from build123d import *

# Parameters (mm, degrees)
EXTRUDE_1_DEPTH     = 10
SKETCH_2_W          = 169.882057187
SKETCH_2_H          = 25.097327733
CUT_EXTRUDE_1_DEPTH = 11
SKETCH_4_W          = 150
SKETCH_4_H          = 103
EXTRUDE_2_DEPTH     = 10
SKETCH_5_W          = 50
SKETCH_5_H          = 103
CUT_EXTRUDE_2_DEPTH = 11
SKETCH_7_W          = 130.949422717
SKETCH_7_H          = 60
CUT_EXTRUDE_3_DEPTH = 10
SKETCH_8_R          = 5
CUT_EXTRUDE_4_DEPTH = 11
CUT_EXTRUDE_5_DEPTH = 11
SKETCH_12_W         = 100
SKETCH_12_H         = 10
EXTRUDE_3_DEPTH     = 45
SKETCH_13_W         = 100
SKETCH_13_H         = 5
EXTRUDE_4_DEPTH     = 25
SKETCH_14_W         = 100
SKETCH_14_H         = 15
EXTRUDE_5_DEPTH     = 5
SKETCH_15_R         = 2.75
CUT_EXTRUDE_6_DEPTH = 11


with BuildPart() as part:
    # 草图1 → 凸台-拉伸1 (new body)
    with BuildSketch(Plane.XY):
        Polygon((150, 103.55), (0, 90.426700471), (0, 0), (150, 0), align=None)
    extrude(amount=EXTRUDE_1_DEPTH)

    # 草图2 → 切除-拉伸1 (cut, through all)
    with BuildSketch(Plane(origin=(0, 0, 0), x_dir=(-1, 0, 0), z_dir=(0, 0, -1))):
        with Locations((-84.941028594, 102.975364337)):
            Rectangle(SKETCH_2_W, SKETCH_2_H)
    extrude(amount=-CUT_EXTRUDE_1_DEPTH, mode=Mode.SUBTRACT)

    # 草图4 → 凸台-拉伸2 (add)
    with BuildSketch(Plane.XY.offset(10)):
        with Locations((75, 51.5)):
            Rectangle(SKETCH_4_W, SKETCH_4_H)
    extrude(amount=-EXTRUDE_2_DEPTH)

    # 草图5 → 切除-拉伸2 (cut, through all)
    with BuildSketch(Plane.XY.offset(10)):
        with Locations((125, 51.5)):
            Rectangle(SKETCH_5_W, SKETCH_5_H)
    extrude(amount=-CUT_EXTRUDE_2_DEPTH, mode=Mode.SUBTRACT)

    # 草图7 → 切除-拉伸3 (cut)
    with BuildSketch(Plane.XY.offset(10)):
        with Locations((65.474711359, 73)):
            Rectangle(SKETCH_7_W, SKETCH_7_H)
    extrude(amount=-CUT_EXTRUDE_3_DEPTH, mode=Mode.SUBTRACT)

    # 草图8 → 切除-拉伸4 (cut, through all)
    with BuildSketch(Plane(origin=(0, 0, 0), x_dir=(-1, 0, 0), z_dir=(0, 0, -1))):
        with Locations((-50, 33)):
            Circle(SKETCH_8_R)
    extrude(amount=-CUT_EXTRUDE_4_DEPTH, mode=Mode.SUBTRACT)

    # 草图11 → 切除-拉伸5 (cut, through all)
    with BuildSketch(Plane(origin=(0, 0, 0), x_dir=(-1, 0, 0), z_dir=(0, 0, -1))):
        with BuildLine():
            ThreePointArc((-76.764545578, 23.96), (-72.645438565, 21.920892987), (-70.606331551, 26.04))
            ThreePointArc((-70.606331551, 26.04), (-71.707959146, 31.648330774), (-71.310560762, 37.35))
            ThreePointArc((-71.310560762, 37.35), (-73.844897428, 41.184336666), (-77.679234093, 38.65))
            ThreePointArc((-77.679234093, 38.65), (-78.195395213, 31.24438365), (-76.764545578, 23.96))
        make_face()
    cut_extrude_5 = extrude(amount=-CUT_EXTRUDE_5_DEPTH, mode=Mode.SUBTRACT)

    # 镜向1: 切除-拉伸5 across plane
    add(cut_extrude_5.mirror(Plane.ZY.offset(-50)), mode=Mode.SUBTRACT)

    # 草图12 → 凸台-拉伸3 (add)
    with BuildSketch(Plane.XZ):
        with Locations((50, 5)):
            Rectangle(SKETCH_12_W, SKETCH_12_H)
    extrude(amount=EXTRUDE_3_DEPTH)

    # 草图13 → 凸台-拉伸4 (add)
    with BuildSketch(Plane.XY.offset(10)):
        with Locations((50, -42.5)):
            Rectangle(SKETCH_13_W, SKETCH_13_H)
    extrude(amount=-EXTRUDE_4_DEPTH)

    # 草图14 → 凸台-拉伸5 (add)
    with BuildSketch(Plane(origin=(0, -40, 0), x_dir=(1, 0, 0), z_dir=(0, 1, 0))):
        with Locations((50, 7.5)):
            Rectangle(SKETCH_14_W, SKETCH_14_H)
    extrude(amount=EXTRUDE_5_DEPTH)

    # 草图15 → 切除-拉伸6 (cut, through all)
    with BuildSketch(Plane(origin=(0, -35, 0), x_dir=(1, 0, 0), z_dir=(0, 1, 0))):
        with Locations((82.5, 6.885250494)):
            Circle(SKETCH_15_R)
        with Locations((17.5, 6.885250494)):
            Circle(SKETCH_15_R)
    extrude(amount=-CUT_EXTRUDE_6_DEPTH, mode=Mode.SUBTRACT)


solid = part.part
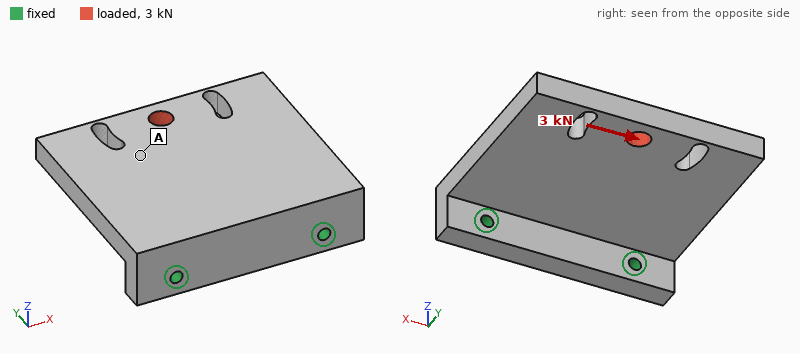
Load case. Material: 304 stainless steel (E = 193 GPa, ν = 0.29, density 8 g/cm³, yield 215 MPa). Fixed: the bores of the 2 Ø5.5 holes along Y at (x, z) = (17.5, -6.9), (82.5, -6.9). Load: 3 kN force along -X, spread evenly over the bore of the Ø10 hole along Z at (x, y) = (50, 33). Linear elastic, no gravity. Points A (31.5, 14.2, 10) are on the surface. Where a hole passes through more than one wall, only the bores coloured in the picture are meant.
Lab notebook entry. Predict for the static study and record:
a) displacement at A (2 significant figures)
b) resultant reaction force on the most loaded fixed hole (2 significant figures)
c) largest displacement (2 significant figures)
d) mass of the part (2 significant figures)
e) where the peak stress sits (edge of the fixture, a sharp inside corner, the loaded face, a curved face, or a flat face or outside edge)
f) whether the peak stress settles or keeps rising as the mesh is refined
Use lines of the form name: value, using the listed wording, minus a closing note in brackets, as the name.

displacement at A: 13 µm
resultant reaction force on the most loaded fixed hole: 3.5 kN
largest displacement: 26 µm
mass of the part: 790 g
where the peak stress sits: edge of the fixture
whether the peak stress settles or keeps rising as the mesh is refined: keeps rising
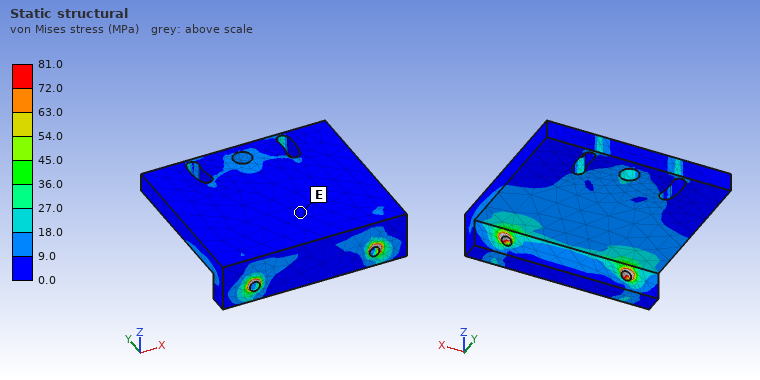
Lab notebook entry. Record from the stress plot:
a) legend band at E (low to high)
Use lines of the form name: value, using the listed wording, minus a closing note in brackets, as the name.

legend band at E: 0.0 to 9.0 MPa
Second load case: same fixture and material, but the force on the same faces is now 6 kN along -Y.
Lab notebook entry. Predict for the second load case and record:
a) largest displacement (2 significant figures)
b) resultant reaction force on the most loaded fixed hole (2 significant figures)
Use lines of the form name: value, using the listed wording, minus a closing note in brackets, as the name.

largest displacement: 53 µm
resultant reaction force on the most loaded fixed hole: 3.0 kN
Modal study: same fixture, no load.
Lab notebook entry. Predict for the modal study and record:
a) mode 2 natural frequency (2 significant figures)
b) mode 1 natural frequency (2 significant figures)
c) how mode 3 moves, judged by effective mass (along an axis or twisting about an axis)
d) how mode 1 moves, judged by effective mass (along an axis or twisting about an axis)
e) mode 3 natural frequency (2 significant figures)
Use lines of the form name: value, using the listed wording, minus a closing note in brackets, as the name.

mode 2 natural frequency: 2100 Hz
mode 1 natural frequency: 890 Hz
how mode 3 moves, judged by effective mass: along X
how mode 1 moves, judged by effective mass: along Z
mode 3 natural frequency: 3800 Hz
